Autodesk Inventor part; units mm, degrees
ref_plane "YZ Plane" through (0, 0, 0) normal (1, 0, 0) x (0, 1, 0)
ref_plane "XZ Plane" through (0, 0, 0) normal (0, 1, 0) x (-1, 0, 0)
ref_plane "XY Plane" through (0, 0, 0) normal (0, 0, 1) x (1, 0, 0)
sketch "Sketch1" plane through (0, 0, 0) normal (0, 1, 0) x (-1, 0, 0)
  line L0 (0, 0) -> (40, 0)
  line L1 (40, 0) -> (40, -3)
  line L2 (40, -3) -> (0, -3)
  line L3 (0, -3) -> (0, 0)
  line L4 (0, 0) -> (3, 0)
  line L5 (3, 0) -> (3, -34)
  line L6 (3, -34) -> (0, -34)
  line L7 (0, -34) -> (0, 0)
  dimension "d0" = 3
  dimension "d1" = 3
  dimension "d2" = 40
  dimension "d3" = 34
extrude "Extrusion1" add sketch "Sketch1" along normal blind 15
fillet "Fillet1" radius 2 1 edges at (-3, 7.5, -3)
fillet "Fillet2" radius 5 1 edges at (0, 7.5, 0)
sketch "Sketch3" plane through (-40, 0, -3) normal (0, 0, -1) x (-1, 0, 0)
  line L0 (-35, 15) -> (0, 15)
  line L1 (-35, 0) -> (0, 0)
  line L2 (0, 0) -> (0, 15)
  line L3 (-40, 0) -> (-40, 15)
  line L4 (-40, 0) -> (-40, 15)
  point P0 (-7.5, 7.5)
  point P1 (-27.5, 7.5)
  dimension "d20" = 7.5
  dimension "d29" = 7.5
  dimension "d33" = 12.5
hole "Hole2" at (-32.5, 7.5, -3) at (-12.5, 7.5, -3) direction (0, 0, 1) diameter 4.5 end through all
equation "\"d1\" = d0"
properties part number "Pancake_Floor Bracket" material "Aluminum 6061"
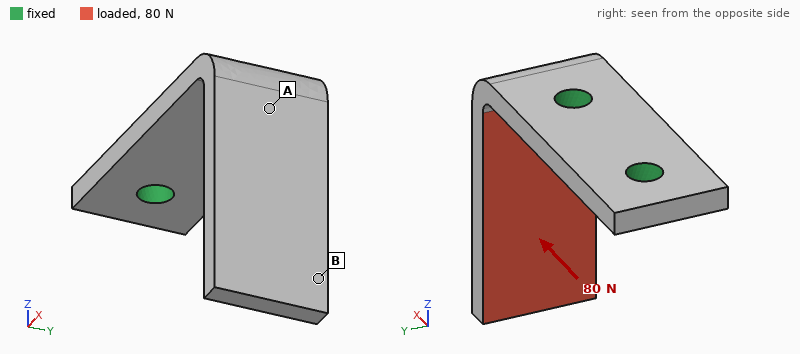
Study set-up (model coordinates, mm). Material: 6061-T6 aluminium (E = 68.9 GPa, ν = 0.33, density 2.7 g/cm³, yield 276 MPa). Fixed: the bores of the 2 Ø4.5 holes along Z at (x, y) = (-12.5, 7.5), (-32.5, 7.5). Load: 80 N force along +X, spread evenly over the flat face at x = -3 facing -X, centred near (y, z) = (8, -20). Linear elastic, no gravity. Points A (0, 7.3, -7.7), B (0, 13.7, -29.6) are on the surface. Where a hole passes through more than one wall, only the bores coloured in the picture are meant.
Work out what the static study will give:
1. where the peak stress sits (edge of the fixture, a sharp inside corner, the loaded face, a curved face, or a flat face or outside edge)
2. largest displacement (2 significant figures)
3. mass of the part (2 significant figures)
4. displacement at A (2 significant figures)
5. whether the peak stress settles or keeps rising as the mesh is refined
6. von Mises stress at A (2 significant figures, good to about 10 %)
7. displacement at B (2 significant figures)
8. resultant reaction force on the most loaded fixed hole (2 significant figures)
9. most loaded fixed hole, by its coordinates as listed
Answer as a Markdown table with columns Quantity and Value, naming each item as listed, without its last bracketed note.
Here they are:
| Quantity | Value |
|---|---|
| where the peak stress sits | edge of the fixture |
| largest displacement | 0.33 mm |
| mass of the part | 8.2 g |
| displacement at A | 0.059 mm |
| whether the peak stress settles or keeps rising as the mesh is refined | keeps rising |
| von Mises stress at A | 38 MPa |
| displacement at B | 0.28 mm |
| resultant reaction force on the most loaded fixed hole | 75 N |
| most loaded fixed hole, by its coordinates as listed | (-12.5, 7.5) |
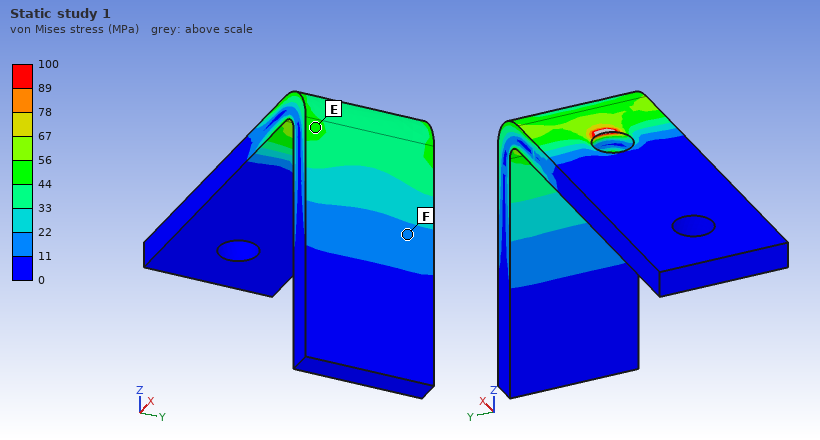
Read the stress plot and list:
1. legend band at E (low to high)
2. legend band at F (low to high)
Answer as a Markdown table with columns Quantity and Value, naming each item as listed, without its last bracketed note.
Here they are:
| Quantity | Value |
|---|---|
| legend band at E | 44 to 56 MPa |
| legend band at F | 11 to 22 MPa |
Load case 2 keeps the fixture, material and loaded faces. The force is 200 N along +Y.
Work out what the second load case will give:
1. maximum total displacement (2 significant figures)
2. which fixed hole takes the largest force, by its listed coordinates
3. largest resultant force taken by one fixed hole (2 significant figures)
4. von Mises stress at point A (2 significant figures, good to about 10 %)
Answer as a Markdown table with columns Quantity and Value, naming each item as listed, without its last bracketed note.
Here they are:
| Quantity | Value |
|---|---|
| maximum total displacement | 0.31 mm |
| which fixed hole takes the largest force, by its listed coordinates | (-12.5, 7.5) |
| largest resultant force taken by one fixed hole | 250 N |
| von Mises stress at point A | 22 MPa |
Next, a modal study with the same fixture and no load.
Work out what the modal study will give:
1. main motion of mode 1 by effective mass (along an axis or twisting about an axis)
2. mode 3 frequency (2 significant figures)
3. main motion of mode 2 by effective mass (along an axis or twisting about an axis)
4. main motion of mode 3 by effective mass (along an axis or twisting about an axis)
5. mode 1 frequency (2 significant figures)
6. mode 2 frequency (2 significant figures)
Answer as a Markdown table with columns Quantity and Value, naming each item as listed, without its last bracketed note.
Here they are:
| Quantity | Value |
|---|---|
| main motion of mode 1 by effective mass | along X |
| mode 3 frequency | 7800 Hz |
| main motion of mode 2 by effective mass | along Y |
| main motion of mode 3 by effective mass | along Z |
| mode 1 frequency | 1600 Hz |
| mode 2 frequency | 2600 Hz |
